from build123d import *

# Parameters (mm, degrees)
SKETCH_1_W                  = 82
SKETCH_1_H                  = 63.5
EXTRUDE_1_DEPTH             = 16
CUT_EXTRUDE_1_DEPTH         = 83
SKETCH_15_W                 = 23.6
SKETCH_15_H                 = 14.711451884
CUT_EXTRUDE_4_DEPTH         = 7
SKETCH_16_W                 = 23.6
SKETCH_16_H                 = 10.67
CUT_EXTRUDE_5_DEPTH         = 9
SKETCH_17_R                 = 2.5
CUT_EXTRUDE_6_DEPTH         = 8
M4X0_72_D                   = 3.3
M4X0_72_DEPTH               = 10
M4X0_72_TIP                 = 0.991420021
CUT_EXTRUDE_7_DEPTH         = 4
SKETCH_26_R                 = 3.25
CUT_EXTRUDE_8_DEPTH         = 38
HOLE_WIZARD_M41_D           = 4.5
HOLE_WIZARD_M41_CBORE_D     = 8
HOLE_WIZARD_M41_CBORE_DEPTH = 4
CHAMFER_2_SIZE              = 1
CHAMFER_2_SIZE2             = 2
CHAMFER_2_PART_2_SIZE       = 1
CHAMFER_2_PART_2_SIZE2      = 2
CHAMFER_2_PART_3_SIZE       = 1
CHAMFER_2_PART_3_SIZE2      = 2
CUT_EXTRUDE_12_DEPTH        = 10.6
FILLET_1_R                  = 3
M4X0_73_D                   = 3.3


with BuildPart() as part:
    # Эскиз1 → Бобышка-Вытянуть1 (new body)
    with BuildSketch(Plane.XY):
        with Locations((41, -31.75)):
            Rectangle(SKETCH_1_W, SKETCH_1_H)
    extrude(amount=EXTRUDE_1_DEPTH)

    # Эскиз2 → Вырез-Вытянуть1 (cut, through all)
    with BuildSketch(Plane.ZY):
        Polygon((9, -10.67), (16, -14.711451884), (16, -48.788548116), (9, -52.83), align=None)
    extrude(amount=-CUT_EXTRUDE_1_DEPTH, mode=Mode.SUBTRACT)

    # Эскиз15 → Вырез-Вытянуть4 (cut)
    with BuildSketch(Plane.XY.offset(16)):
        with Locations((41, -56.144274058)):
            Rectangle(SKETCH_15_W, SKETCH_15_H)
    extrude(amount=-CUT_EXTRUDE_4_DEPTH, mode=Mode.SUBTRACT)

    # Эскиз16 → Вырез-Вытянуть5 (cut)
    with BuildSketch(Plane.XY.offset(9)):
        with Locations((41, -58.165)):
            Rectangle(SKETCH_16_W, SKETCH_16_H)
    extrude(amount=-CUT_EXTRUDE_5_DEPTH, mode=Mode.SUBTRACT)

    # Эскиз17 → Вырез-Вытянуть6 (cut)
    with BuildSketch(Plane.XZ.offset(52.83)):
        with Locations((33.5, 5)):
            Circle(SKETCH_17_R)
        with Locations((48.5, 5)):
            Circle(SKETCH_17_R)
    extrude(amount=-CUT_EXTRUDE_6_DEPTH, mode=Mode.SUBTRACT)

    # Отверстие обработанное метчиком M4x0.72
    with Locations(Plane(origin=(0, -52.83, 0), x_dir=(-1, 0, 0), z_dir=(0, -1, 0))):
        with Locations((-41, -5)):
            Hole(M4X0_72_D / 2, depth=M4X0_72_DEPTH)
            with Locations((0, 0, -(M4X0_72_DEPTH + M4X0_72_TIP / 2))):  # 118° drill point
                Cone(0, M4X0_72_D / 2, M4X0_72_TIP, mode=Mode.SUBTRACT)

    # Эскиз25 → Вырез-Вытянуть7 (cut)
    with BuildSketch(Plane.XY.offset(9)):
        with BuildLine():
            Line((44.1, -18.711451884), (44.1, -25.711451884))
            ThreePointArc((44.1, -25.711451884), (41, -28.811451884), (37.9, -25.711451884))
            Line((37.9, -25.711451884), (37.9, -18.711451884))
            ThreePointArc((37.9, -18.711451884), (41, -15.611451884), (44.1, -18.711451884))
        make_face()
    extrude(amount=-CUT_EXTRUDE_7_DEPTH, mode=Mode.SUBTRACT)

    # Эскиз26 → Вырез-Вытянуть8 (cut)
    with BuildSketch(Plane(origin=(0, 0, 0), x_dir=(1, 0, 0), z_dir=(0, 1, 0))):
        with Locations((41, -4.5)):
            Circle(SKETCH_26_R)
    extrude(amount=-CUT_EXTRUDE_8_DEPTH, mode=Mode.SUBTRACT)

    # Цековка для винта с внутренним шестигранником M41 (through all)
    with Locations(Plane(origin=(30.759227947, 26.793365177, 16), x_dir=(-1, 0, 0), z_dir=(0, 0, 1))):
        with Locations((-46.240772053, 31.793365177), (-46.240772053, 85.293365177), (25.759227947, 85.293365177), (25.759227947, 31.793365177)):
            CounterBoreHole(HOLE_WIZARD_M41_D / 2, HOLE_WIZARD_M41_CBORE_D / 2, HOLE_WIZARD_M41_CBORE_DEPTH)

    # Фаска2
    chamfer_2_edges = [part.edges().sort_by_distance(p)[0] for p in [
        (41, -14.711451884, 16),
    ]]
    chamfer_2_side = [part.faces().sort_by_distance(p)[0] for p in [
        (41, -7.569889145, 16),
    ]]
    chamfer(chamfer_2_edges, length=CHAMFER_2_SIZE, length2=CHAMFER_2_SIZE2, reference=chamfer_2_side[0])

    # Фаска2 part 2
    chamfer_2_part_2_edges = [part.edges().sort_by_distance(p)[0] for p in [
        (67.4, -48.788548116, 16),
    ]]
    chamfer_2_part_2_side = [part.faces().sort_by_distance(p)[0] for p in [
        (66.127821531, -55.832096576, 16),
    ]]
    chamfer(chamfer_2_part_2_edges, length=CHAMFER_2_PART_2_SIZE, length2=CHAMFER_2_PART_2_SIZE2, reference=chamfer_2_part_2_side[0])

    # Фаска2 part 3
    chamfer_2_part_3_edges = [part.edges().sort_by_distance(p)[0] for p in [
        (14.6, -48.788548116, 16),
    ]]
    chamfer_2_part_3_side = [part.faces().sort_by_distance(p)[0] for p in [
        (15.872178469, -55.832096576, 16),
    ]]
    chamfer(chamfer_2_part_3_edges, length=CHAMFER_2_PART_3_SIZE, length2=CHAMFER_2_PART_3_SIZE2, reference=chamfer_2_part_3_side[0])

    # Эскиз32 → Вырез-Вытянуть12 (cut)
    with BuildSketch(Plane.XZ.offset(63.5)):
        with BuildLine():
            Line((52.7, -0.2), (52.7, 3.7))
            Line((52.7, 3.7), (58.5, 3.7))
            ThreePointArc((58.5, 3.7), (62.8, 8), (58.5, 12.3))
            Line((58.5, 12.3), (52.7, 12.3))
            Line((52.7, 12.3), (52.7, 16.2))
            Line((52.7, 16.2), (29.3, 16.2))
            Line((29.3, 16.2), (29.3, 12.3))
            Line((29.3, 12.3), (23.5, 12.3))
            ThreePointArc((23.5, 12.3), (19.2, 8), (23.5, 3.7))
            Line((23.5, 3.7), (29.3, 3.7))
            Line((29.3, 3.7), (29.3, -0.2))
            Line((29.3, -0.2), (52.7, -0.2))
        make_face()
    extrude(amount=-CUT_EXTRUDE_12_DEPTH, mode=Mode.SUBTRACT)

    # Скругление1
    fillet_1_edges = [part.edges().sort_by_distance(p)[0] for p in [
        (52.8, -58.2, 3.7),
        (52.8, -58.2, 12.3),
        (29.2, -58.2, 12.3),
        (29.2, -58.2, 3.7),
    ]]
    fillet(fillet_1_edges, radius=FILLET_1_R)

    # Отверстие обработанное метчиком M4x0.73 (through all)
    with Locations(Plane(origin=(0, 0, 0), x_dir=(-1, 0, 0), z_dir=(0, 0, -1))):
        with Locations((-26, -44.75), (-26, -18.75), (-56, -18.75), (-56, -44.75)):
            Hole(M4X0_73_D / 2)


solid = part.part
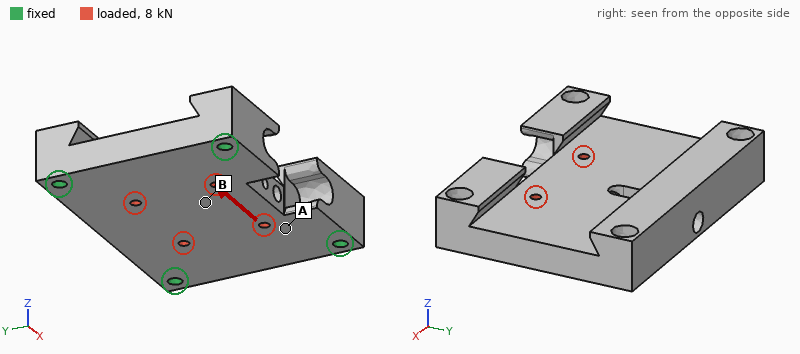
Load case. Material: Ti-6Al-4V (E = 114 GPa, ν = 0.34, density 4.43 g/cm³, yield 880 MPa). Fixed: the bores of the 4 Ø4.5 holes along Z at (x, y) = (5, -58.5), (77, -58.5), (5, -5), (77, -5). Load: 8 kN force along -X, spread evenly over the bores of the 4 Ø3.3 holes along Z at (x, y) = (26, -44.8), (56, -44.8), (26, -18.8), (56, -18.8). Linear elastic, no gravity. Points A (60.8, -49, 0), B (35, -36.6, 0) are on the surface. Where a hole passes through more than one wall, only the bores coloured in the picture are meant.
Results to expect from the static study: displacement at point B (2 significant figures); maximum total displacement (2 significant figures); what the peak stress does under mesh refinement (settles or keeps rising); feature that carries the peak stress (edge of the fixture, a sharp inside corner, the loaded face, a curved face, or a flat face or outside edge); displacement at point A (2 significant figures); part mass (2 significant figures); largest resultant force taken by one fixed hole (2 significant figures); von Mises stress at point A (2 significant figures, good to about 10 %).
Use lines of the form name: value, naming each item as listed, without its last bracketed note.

displacement at point B: 3.6 µm
maximum total displacement: 4.9 µm
what the peak stress does under mesh refinement: keeps rising
feature that carries the peak stress: a sharp inside corner
displacement at point A: 3.5 µm
part mass: 230 g
largest resultant force taken by one fixed hole: 2.4 kN
von Mises stress at point A: 12 MPa
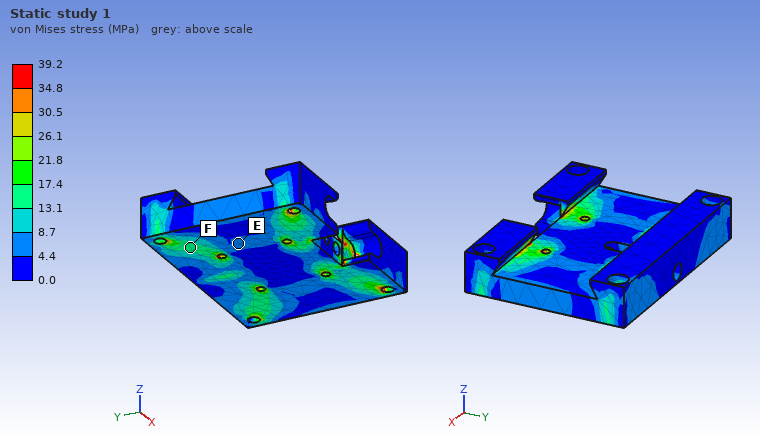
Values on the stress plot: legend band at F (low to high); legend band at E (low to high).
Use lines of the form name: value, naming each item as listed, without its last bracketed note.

legend band at F: 13.1 to 17.4 MPa
legend band at E: 4.4 to 8.7 MPa
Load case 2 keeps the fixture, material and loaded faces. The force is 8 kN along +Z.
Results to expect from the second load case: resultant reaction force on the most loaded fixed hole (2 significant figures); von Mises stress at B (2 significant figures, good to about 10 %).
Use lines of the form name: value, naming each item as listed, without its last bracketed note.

resultant reaction force on the most loaded fixed hole: 2.2 kN
von Mises stress at B: 34 MPa
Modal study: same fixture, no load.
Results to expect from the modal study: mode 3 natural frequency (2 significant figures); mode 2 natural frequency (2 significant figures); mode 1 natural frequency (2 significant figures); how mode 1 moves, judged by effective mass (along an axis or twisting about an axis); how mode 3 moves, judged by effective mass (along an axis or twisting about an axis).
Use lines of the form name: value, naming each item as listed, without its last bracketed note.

mode 3 natural frequency: 14 kHz
mode 2 natural frequency: 12 kHz
mode 1 natural frequency: 8100 Hz
how mode 1 moves, judged by effective mass: along Z
how mode 3 moves, judged by effective mass: twisting about Y
